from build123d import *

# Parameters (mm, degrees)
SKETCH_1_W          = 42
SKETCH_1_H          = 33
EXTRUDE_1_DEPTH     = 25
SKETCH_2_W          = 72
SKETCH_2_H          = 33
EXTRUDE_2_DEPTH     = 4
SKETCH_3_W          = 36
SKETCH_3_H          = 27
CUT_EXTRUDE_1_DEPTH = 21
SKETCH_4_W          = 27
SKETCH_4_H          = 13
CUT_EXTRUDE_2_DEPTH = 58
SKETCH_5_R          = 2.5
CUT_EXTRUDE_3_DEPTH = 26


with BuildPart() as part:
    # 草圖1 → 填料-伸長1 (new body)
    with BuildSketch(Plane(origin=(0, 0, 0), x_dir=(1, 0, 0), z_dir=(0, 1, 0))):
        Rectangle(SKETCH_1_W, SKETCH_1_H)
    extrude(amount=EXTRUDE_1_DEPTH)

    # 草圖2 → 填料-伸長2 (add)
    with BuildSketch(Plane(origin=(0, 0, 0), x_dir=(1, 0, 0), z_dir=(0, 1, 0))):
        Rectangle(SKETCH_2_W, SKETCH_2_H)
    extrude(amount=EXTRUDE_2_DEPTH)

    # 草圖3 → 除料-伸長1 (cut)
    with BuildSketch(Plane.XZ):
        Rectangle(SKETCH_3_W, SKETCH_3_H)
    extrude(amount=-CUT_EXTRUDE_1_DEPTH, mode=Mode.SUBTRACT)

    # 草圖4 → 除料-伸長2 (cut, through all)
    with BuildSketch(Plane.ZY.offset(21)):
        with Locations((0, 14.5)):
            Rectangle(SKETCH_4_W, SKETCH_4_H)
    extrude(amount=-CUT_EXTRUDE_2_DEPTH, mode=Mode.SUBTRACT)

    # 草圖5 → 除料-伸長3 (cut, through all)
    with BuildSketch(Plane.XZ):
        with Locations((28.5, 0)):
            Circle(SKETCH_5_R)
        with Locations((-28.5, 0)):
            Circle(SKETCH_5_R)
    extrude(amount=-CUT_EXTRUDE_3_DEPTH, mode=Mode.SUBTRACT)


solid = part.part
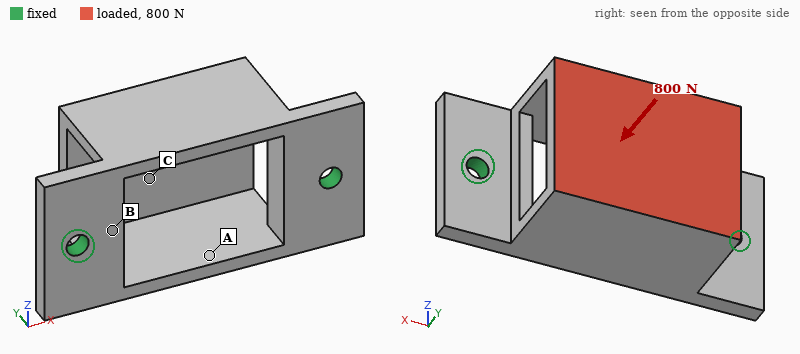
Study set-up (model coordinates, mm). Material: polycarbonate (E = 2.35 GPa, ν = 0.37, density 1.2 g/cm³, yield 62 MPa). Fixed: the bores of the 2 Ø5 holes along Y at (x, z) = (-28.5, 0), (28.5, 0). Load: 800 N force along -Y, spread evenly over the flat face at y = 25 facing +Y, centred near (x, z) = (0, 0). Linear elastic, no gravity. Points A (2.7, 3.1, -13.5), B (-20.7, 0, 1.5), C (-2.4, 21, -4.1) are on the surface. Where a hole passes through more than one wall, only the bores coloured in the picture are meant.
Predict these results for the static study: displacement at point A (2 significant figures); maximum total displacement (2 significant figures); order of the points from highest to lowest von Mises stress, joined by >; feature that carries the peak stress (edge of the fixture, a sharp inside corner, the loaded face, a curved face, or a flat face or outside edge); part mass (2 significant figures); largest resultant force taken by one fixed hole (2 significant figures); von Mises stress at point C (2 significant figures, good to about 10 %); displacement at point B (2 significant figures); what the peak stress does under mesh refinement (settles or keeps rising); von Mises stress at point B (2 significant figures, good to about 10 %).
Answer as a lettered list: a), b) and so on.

a) 0.59 mm
b) 0.94 mm
c) B > C > A
d) edge of the fixture
e) 19 g
f) 450 N
g) 13 MPa
h) 0.17 mm
i) keeps rising
j) 23 MPa
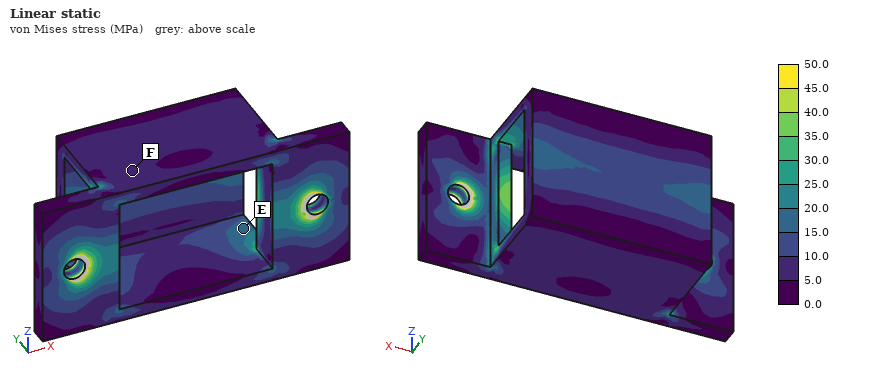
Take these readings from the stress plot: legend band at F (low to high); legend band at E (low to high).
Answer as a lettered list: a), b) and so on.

a) 5.0 to 10.0 MPa
b) 15.0 to 20.0 MPa
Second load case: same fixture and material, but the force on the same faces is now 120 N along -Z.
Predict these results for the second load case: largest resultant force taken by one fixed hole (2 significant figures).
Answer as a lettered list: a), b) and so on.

a) 60 N
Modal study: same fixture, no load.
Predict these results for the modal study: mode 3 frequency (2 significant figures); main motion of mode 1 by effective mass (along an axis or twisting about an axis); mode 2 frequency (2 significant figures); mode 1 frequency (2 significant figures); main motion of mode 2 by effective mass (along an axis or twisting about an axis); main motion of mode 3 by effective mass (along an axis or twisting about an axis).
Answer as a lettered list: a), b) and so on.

a) 1700 Hz
b) along Z
c) 1500 Hz
d) 650 Hz
e) along Y
f) along X
